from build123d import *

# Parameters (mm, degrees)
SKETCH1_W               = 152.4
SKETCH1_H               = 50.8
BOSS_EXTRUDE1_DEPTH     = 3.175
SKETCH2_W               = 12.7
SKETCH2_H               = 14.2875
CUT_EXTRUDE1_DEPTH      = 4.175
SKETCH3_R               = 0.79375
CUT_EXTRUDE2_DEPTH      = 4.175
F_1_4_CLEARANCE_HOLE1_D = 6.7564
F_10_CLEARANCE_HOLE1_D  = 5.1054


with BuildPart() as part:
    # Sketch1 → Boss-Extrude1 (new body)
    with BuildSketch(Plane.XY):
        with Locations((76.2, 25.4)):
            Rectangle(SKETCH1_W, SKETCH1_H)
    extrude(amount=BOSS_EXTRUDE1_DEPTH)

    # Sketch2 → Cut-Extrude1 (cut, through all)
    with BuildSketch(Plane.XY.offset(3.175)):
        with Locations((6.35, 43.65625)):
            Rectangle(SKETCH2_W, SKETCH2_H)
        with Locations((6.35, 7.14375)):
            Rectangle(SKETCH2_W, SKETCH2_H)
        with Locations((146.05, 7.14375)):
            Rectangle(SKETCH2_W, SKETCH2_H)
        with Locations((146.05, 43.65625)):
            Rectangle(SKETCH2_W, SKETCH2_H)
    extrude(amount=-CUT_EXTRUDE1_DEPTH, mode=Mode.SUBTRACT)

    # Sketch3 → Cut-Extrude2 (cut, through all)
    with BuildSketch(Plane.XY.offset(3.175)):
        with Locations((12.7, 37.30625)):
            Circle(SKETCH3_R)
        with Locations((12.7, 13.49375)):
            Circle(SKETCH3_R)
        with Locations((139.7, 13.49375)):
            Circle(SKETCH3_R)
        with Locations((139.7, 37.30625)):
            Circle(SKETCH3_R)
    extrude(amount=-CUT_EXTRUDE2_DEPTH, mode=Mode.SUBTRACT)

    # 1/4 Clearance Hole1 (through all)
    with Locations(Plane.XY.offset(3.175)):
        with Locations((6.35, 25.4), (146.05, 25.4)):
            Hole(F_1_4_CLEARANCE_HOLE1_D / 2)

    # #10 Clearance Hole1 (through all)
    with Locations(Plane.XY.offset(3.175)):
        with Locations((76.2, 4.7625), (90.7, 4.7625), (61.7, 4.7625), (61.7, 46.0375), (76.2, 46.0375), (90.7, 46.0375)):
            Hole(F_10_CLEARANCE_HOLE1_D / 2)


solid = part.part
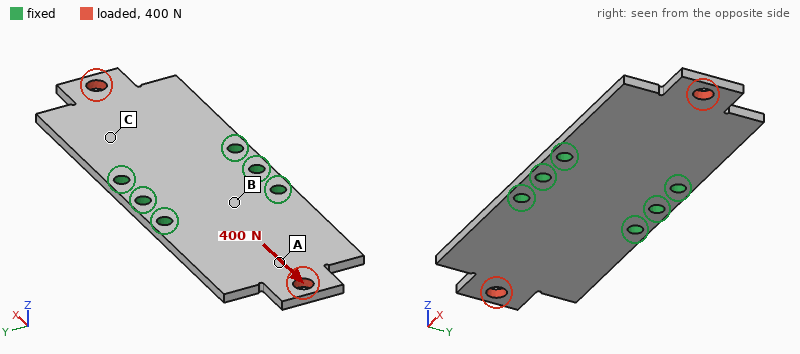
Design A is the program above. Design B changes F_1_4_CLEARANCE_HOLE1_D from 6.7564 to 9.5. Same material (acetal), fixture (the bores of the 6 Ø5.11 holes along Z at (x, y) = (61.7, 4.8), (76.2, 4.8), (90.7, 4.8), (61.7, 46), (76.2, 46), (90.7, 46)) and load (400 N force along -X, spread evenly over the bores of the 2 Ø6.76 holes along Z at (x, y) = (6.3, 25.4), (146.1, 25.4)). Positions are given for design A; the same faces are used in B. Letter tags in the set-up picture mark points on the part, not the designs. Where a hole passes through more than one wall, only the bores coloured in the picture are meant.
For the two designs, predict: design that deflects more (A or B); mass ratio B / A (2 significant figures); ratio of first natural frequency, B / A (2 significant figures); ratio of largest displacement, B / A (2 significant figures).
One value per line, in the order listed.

B
0.99
1.0
1.3
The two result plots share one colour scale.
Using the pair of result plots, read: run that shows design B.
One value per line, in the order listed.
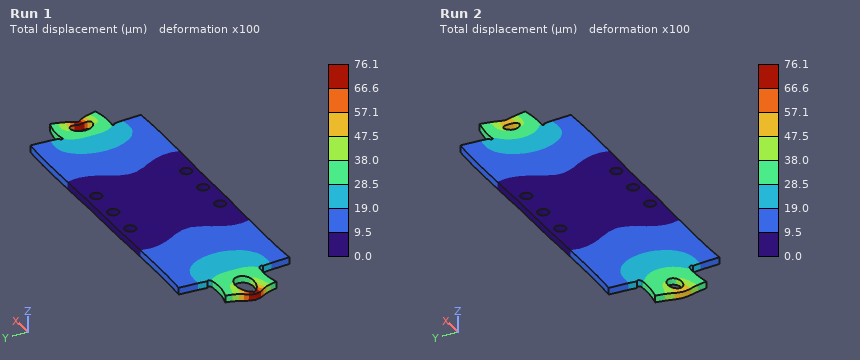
Run 1
